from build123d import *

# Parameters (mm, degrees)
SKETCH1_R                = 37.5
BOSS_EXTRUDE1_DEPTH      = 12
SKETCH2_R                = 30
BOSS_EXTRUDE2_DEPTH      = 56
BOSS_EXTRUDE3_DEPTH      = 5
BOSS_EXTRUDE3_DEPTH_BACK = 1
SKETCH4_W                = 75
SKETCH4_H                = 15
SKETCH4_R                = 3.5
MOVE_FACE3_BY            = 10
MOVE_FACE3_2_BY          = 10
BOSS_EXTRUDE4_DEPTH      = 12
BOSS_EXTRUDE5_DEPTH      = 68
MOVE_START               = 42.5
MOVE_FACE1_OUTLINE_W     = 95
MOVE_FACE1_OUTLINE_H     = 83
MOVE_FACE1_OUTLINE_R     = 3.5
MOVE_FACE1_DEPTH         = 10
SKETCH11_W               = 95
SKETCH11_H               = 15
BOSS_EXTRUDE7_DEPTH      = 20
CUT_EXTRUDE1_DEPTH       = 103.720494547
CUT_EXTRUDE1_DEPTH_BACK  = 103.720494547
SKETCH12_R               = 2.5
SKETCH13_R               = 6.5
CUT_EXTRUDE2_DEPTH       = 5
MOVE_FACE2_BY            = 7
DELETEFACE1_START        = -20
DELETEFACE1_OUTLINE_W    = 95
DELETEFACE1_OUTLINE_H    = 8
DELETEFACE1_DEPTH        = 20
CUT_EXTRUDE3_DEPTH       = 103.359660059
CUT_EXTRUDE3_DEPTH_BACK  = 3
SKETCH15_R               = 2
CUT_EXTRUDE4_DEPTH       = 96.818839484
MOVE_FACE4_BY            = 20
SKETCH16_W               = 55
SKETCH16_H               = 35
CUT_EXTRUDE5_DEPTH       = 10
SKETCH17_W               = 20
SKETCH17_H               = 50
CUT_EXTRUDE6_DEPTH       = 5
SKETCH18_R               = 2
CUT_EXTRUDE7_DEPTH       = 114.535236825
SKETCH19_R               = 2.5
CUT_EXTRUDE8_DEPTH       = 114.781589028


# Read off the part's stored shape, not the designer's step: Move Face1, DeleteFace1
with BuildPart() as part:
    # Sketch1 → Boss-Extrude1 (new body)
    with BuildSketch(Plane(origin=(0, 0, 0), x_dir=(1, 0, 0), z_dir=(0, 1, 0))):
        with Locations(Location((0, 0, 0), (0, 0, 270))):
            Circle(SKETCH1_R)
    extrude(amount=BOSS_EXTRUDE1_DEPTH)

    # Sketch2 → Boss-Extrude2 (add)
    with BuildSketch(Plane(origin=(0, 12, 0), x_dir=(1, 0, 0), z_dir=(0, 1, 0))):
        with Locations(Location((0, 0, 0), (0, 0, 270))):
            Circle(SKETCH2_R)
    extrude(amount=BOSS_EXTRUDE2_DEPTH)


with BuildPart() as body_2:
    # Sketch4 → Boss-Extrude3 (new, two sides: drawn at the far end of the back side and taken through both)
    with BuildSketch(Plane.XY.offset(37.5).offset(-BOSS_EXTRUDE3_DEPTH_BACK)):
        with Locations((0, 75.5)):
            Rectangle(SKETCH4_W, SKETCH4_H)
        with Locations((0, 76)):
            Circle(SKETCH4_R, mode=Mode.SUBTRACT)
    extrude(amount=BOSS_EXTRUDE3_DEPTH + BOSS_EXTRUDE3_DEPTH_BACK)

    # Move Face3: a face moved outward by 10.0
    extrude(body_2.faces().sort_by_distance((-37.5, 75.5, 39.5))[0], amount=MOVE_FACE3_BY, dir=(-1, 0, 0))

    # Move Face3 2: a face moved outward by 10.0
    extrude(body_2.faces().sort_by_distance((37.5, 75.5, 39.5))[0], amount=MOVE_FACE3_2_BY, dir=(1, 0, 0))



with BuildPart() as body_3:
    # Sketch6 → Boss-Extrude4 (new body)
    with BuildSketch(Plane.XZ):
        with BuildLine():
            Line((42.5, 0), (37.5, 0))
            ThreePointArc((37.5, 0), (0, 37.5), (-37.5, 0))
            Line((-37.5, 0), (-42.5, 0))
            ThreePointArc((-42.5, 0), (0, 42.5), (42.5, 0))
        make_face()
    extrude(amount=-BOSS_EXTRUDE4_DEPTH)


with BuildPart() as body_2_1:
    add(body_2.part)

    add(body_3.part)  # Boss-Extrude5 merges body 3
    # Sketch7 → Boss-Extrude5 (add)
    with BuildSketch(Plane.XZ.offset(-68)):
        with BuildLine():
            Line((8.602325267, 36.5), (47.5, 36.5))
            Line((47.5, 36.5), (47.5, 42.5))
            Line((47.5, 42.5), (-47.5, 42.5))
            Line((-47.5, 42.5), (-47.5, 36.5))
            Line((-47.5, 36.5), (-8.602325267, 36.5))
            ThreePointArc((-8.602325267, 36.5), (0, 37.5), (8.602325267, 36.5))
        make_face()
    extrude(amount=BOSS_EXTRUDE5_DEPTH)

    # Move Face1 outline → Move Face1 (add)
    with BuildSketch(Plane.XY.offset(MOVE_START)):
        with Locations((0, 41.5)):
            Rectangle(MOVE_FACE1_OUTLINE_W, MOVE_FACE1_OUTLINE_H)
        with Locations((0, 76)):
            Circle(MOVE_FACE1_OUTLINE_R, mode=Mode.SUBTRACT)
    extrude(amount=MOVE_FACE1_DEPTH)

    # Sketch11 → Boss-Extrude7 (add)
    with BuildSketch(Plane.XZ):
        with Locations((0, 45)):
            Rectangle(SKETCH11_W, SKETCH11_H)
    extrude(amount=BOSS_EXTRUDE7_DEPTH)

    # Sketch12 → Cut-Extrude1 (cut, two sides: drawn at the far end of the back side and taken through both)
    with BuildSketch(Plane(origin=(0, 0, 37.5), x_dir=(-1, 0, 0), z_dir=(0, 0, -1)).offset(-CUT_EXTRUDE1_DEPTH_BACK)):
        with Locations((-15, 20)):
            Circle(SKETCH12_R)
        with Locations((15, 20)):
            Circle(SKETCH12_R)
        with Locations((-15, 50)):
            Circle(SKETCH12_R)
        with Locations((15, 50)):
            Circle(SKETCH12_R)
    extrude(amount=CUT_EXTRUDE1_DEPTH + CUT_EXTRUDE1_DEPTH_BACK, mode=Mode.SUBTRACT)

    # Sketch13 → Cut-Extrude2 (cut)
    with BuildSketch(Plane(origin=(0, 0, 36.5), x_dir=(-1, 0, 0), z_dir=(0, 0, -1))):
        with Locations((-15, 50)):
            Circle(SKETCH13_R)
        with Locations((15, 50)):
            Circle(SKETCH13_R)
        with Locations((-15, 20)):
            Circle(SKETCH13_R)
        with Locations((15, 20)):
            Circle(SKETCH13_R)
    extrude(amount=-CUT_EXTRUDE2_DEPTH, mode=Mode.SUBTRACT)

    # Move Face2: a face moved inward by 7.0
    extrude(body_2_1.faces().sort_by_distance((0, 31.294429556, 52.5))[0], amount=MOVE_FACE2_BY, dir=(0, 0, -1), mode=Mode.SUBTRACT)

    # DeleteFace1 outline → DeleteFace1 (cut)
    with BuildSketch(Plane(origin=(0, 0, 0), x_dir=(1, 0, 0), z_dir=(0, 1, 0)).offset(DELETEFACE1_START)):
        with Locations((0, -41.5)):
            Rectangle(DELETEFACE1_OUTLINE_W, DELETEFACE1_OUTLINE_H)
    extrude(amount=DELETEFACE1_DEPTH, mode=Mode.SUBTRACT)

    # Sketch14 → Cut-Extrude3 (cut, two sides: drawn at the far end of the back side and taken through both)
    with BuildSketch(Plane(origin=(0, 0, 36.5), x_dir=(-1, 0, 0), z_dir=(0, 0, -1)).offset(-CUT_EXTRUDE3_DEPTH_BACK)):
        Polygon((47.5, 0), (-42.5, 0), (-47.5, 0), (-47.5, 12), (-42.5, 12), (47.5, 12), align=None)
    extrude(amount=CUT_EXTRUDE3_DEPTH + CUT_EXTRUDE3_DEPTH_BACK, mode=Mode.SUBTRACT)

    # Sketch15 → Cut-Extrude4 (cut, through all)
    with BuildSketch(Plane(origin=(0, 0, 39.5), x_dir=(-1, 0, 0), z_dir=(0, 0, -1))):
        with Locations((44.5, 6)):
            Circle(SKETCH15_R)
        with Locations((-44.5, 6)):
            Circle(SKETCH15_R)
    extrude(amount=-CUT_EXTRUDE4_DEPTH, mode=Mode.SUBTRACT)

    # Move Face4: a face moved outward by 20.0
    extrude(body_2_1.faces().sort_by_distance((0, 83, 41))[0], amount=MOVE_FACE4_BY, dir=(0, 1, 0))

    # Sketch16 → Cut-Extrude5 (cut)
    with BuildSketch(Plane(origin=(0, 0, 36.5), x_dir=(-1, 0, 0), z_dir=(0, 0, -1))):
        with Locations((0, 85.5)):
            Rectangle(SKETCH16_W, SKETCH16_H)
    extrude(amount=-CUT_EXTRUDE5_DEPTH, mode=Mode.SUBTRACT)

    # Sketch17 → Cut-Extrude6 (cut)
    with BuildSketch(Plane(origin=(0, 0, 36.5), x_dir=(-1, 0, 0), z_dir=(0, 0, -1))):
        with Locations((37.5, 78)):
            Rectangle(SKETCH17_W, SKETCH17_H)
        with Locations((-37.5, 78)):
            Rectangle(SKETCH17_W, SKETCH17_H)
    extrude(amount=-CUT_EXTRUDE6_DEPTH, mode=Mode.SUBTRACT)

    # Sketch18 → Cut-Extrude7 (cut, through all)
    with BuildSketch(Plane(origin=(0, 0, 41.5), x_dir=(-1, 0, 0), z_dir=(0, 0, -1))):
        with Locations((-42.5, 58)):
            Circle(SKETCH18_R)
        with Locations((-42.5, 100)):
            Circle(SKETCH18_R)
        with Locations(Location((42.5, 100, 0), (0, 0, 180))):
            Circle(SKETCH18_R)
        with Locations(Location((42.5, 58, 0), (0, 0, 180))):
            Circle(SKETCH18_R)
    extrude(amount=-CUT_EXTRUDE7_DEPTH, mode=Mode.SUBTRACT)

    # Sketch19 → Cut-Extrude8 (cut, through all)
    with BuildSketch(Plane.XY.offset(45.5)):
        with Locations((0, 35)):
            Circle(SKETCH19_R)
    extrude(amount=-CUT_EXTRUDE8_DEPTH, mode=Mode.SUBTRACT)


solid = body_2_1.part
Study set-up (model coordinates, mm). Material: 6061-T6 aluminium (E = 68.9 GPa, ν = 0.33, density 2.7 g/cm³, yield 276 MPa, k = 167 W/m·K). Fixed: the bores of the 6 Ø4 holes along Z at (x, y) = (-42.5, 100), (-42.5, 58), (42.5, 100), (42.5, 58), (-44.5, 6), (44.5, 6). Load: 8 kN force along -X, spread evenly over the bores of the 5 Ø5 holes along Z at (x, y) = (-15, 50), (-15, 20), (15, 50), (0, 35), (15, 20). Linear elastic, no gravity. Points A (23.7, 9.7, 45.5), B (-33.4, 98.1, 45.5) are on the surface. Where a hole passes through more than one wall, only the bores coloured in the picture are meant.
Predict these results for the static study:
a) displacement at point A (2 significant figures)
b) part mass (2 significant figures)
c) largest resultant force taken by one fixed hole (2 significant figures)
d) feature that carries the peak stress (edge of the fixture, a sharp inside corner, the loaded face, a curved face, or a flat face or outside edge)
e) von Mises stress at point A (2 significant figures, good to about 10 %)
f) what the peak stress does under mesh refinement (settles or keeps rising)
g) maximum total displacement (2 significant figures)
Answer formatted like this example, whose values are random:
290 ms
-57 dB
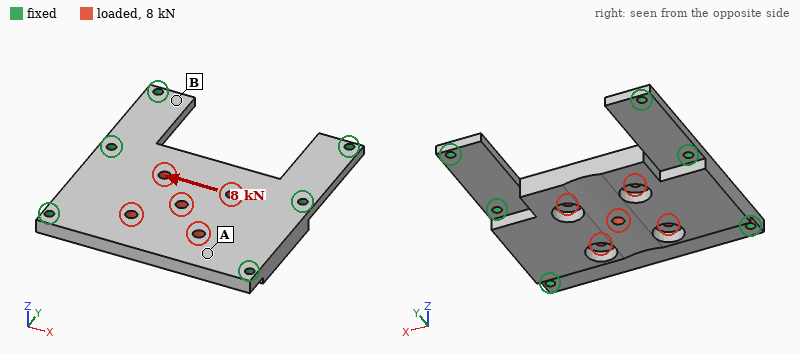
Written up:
6.4 µm
140 g
2.1 kN
edge of the fixture
16 MPa
keeps rising
13 µm
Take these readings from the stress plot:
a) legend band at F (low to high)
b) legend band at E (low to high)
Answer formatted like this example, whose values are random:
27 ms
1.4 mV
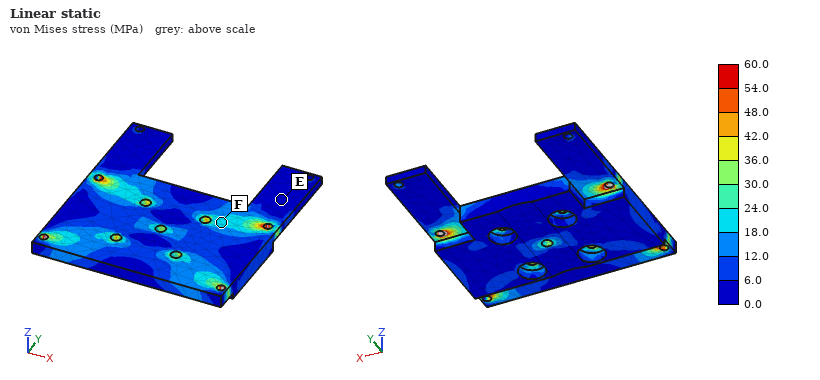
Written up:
18.0 to 24.0 MPa
0.0 to 6.0 MPa
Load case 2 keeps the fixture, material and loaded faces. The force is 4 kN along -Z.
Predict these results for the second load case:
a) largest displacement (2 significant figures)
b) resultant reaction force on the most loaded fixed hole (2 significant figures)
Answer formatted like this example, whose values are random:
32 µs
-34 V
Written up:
0.15 mm
1.8 kN
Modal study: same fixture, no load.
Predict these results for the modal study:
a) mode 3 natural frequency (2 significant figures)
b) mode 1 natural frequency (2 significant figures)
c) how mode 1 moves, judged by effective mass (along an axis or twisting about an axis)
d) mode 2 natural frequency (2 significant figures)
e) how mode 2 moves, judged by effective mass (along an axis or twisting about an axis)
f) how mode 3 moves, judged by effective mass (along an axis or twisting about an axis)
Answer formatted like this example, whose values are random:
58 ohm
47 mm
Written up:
8900 Hz
3400 Hz
along Z
5500 Hz
twisting about X
twisting about Y
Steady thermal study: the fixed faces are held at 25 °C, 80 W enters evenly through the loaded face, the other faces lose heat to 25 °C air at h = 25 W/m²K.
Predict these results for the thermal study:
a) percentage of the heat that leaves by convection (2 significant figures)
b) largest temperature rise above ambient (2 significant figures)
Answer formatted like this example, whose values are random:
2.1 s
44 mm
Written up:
7.9 %
28 K
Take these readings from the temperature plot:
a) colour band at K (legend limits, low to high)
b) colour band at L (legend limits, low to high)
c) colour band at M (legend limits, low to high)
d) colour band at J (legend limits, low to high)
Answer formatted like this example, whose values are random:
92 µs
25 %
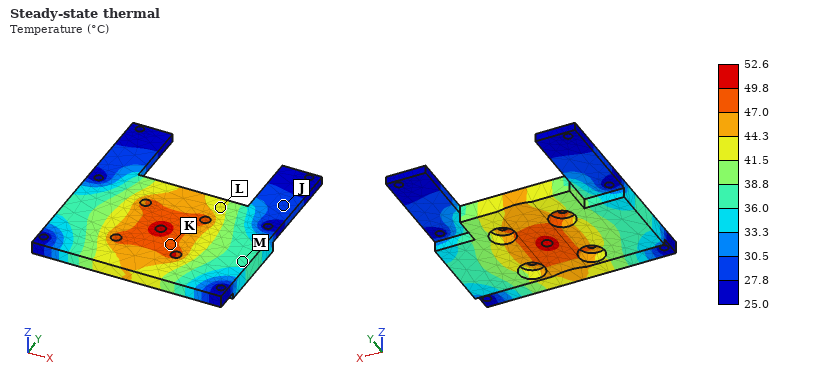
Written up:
47.0 to 49.8 °C
41.5 to 44.3 °C
36.0 to 38.8 °C
27.8 to 30.5 °C
